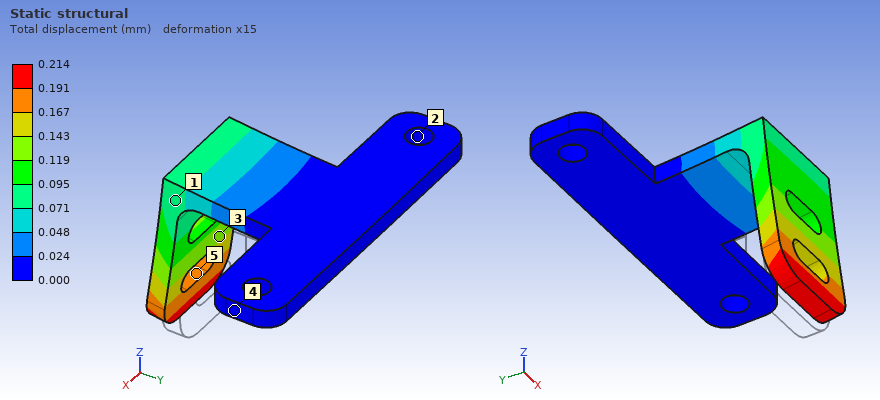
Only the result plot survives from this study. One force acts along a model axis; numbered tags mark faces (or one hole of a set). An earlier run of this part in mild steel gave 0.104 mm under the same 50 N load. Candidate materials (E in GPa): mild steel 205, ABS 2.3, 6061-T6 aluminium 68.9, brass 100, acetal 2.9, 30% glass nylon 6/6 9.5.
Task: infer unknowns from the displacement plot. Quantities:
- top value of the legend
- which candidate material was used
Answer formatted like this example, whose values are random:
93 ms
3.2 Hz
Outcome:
0.214 mm
brass
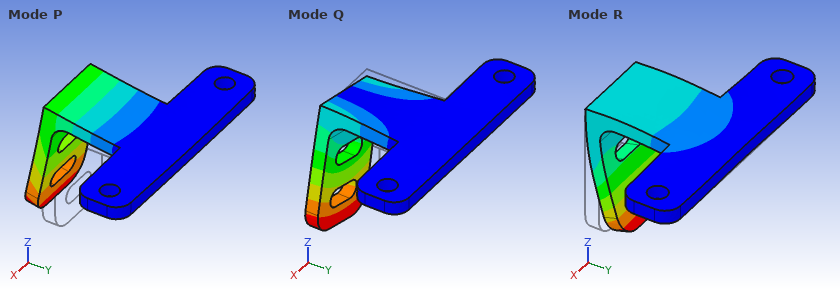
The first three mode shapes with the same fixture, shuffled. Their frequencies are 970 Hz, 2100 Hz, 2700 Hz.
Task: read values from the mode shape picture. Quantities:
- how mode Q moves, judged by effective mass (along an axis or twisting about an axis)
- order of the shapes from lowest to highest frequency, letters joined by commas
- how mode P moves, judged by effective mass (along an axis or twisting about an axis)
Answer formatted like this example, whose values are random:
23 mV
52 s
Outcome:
along X
P, Q, R
along Z
